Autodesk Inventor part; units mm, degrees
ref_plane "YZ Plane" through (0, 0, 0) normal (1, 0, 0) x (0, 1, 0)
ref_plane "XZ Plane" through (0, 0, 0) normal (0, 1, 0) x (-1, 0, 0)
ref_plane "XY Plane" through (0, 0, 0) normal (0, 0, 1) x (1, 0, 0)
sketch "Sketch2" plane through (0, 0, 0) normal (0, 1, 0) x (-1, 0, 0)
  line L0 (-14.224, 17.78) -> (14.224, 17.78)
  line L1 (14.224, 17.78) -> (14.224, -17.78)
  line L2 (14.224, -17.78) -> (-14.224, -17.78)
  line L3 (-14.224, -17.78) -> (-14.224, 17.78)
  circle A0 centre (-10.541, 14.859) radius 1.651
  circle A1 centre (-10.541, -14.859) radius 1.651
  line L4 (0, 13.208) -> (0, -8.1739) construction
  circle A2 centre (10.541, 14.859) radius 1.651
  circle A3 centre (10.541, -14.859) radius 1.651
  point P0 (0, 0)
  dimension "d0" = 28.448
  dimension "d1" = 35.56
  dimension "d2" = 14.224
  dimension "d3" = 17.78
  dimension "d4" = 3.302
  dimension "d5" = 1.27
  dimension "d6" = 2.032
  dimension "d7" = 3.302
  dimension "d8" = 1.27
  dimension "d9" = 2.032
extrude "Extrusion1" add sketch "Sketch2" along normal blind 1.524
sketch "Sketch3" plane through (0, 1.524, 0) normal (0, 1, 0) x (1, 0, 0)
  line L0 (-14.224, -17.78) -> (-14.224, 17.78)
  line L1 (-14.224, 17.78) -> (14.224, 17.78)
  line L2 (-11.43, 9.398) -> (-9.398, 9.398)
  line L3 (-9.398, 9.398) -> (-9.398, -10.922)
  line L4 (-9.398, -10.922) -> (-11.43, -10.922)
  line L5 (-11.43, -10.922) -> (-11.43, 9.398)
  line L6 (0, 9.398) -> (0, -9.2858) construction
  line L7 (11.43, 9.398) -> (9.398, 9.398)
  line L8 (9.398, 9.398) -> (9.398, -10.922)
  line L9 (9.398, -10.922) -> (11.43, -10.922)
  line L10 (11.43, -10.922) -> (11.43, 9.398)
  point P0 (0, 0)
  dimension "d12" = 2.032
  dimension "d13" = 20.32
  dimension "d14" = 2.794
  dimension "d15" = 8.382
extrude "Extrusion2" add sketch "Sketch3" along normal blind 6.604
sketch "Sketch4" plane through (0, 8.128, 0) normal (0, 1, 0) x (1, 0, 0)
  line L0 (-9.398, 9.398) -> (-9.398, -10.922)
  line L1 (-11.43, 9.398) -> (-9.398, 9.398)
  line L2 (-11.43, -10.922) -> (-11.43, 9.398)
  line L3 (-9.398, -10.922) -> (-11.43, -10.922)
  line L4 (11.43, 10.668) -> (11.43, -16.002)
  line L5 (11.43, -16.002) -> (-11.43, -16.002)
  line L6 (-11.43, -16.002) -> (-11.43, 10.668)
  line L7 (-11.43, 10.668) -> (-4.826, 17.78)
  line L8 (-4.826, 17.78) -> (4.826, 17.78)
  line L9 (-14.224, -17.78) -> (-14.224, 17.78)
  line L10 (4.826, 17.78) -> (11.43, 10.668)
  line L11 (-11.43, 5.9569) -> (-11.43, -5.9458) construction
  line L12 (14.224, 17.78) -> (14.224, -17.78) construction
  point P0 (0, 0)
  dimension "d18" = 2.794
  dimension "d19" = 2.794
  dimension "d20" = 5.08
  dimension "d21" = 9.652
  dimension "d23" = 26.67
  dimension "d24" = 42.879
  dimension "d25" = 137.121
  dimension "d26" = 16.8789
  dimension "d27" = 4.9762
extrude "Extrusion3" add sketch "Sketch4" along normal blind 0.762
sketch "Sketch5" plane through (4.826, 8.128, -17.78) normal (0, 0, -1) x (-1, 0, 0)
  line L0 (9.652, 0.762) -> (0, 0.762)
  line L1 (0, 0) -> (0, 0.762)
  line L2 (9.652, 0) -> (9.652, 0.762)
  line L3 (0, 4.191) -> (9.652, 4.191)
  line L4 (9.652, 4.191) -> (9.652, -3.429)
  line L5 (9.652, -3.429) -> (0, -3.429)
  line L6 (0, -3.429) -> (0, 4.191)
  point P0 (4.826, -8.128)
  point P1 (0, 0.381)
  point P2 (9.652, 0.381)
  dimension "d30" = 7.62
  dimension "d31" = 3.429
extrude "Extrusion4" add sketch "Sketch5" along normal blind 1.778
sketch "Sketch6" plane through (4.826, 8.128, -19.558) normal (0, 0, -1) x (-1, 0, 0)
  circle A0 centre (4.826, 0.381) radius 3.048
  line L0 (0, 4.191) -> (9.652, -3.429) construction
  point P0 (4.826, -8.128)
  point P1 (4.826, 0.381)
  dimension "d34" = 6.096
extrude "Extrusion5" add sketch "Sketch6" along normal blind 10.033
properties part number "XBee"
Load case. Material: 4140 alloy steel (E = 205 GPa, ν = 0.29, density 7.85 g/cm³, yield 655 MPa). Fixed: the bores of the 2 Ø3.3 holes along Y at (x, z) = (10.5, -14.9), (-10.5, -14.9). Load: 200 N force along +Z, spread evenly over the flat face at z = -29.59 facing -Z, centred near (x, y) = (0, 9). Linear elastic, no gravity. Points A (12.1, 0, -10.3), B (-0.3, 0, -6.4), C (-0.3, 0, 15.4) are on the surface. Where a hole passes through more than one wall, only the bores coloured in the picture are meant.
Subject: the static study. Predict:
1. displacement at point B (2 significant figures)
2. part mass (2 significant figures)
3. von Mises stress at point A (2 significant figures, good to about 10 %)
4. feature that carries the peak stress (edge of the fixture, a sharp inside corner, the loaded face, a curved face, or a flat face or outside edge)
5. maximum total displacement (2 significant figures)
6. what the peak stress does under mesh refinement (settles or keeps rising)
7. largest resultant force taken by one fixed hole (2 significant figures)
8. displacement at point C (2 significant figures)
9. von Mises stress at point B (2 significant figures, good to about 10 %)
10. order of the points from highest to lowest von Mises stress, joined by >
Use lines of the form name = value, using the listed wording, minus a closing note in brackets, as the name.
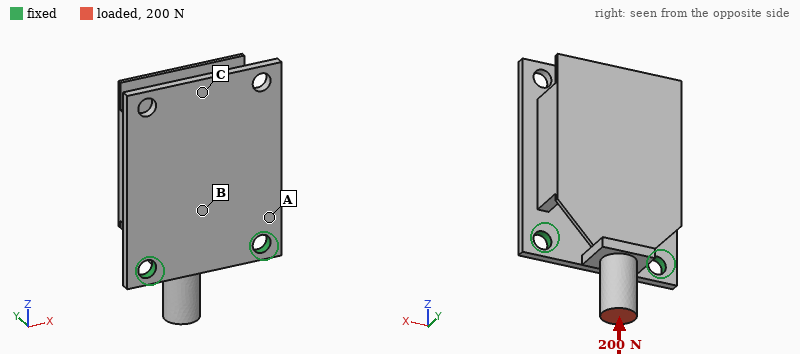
displacement at point B = 0.033 mm
part mass = 24 g
von Mises stress at point A = 170 MPa
feature that carries the peak stress = edge of the fixture
maximum total displacement = 0.20 mm
what the peak stress does under mesh refinement = keeps rising
largest resultant force taken by one fixed hole = 100 N
displacement at point C = 0.18 mm
von Mises stress at point B = 53 MPa
order of the points from highest to lowest von Mises stress, joined by > = A > B > C
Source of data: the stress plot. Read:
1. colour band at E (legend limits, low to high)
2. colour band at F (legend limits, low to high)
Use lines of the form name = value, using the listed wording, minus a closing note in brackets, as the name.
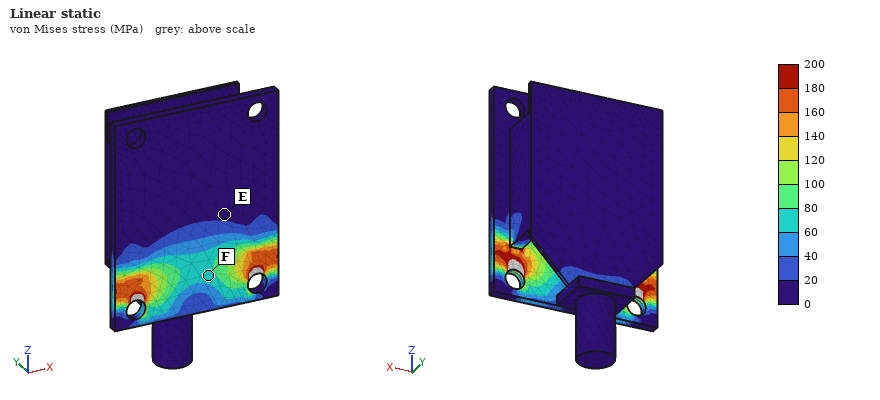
colour band at E = 0 to 20 MPa
colour band at F = 60 to 80 MPa
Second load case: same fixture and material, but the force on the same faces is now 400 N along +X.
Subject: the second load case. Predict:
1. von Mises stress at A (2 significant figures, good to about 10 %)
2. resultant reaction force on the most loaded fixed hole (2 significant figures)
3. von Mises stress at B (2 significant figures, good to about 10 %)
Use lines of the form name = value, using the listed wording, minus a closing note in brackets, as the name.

von Mises stress at A = 150 MPa
resultant reaction force on the most loaded fixed hole = 370 N
von Mises stress at B = 66 MPa
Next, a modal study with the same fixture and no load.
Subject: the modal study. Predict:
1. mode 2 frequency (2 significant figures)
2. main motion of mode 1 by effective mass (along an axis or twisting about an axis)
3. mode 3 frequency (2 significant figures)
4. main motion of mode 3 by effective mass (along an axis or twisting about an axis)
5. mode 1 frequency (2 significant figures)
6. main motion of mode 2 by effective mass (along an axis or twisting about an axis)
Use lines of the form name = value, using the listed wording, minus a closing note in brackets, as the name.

mode 2 frequency = 1200 Hz
main motion of mode 1 by effective mass = twisting about X
mode 3 frequency = 3500 Hz
main motion of mode 3 by effective mass = along X
mode 1 frequency = 790 Hz
main motion of mode 2 by effective mass = along Y
